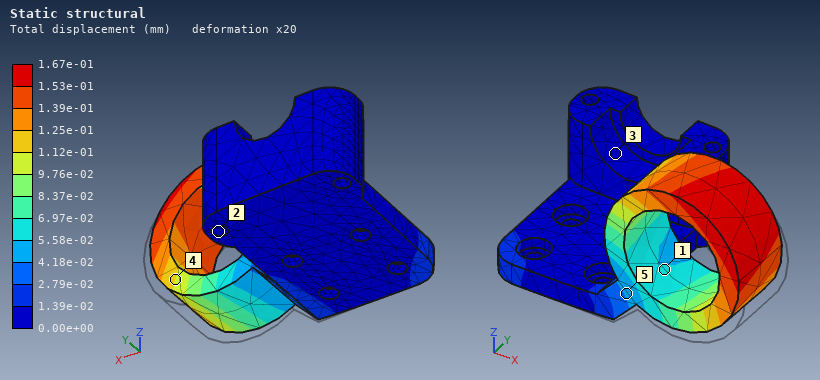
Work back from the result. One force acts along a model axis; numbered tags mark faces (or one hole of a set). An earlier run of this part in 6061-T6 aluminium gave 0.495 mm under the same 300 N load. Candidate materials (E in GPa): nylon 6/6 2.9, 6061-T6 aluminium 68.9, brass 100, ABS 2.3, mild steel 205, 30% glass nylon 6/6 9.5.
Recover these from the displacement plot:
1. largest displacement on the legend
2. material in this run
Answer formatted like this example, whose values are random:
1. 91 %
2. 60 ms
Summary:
1. 1.67e-01 mm
2. mild steel
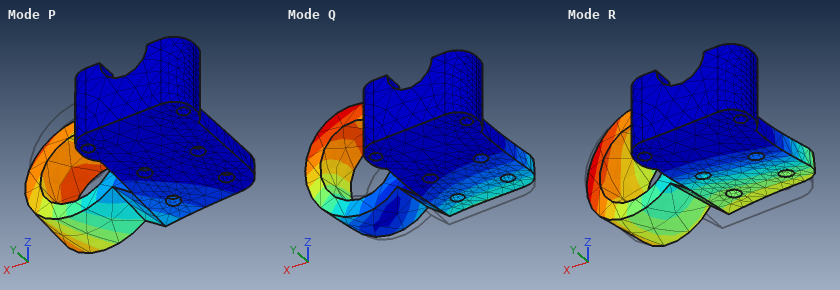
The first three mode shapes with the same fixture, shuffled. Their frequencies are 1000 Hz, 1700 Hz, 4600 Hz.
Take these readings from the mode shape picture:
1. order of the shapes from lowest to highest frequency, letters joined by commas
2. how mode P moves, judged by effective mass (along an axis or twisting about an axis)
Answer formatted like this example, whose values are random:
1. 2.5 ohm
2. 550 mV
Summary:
1. P, Q, R
2. along Z
